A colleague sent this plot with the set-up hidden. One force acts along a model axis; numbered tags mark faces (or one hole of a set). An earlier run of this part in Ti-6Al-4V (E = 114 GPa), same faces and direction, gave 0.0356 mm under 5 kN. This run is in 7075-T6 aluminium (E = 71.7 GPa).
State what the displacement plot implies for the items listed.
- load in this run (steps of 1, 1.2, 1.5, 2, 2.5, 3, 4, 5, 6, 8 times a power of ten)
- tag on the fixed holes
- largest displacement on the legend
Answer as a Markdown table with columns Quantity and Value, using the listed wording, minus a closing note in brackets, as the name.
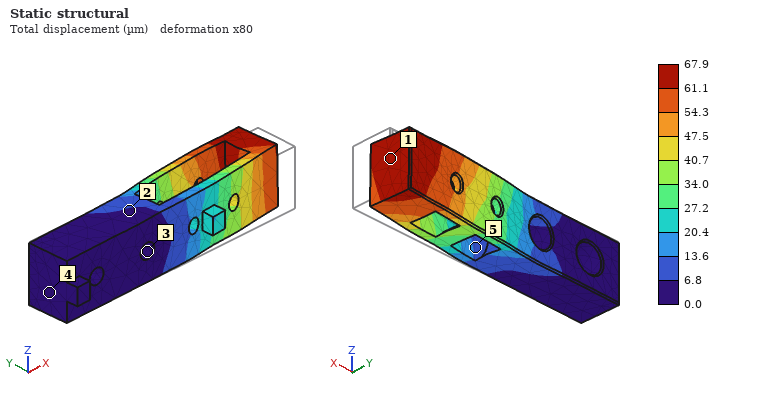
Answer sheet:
| Quantity | Value |
|---|---|
| load in this run | 6 kN |
| tag on the fixed holes | 3 |
| largest displacement on the legend | 67.9 µm |
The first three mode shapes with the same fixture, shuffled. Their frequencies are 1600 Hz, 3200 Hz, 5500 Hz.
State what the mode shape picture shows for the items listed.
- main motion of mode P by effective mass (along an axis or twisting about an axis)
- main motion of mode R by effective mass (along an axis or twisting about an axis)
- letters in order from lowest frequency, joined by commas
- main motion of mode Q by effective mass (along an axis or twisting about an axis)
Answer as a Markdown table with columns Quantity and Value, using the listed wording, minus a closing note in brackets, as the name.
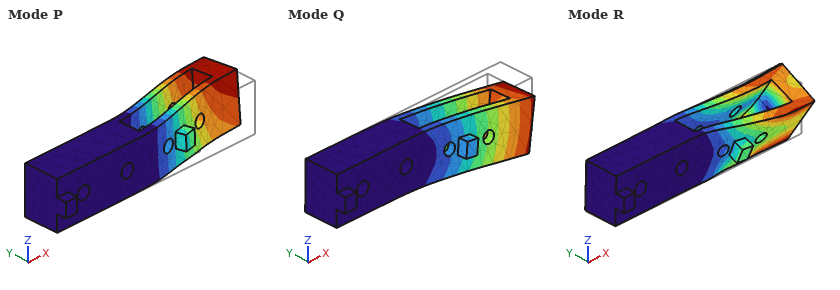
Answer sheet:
| Quantity | Value |
|---|---|
| main motion of mode P by effective mass | along Y |
| main motion of mode R by effective mass | twisting about X |
| letters in order from lowest frequency, joined by commas | P, Q, R |
| main motion of mode Q by effective mass | along Z |
